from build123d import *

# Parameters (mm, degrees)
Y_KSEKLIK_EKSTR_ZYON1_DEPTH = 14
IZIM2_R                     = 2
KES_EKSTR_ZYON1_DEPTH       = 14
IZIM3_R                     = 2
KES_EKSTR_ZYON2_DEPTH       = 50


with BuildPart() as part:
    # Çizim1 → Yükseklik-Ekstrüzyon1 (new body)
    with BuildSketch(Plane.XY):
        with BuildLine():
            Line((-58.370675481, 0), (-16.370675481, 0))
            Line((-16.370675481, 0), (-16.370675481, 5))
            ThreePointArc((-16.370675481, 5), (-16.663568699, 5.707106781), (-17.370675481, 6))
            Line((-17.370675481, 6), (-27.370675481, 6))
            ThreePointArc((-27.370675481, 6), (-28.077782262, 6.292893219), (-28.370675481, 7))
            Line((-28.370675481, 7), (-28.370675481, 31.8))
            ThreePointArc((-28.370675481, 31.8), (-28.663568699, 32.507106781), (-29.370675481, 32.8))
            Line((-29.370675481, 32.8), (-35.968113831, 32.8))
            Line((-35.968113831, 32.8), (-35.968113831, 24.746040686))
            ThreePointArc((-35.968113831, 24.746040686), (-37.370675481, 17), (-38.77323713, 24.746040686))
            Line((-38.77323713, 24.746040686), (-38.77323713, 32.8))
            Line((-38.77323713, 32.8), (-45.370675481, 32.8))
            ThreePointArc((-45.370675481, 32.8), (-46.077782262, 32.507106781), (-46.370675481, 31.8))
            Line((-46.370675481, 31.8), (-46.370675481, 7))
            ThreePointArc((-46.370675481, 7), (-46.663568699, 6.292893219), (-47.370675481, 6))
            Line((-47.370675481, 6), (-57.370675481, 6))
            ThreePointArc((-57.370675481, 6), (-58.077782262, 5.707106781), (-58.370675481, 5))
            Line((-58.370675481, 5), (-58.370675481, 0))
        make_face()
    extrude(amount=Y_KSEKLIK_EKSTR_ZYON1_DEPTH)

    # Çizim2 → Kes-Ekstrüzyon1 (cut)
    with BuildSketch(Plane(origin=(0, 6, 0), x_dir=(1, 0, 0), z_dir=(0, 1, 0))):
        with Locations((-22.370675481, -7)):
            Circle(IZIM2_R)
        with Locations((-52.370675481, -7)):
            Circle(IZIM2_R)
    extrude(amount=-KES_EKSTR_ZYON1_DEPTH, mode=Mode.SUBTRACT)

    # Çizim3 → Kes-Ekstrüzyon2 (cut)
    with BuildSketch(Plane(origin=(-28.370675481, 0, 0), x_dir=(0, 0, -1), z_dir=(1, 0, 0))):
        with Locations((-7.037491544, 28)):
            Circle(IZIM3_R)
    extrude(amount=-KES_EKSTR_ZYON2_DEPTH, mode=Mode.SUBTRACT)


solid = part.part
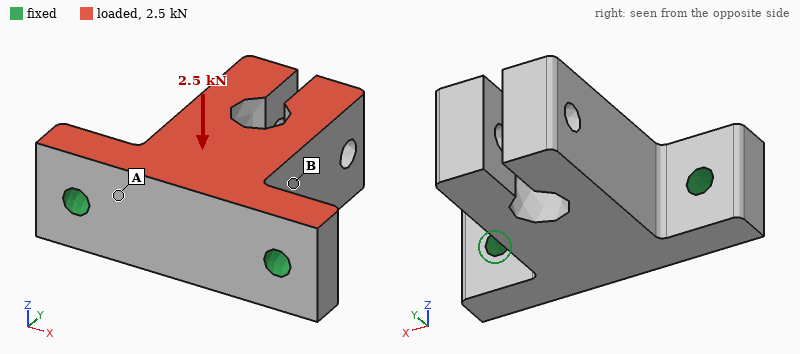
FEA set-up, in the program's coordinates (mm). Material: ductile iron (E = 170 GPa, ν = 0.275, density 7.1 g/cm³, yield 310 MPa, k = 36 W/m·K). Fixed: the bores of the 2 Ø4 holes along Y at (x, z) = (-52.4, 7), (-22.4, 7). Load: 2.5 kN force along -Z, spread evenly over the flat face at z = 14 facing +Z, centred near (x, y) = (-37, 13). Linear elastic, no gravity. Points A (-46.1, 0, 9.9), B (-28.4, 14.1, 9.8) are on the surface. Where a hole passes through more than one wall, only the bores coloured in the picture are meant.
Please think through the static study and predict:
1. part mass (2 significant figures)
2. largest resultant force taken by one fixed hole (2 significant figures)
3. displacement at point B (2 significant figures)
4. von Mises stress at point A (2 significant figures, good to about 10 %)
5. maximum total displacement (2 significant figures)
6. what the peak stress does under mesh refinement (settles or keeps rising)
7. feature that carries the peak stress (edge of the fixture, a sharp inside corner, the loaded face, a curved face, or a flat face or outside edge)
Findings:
63 g
1.3 kN
22 µm
55 MPa
59 µm
keeps rising
edge of the fixture
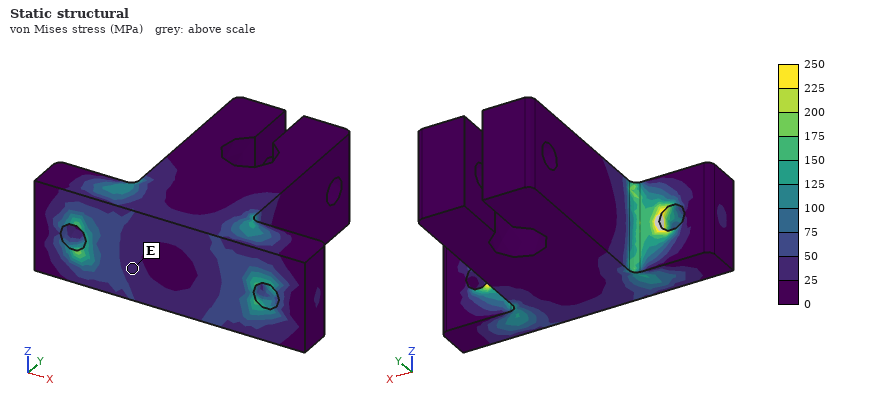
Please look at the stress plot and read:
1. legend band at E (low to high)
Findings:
25 to 50 MPa
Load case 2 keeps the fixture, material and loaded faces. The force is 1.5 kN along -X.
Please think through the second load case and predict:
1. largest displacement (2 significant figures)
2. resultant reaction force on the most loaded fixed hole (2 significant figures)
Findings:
15 µm
1.0 kN
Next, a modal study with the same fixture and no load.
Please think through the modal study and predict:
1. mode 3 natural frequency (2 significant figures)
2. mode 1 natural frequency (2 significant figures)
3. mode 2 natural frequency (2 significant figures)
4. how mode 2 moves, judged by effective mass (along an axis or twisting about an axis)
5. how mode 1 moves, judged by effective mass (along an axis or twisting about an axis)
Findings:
11 kHz
5100 Hz
8900 Hz
along X
along Z
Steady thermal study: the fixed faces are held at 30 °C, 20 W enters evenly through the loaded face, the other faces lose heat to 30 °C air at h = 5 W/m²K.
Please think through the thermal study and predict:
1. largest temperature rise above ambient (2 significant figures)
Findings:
49 K
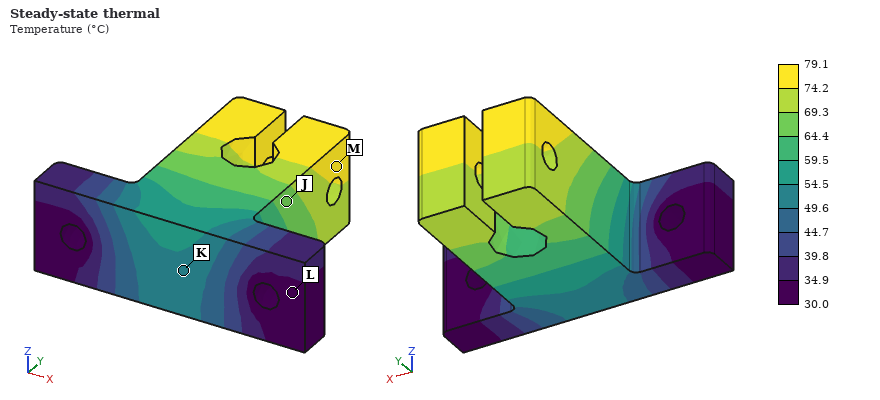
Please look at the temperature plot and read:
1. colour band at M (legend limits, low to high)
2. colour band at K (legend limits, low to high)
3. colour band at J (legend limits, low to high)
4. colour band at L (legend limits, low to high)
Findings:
74.2 to 79.1 °C
49.6 to 54.5 °C
64.4 to 69.3 °C
30.0 to 34.9 °C
